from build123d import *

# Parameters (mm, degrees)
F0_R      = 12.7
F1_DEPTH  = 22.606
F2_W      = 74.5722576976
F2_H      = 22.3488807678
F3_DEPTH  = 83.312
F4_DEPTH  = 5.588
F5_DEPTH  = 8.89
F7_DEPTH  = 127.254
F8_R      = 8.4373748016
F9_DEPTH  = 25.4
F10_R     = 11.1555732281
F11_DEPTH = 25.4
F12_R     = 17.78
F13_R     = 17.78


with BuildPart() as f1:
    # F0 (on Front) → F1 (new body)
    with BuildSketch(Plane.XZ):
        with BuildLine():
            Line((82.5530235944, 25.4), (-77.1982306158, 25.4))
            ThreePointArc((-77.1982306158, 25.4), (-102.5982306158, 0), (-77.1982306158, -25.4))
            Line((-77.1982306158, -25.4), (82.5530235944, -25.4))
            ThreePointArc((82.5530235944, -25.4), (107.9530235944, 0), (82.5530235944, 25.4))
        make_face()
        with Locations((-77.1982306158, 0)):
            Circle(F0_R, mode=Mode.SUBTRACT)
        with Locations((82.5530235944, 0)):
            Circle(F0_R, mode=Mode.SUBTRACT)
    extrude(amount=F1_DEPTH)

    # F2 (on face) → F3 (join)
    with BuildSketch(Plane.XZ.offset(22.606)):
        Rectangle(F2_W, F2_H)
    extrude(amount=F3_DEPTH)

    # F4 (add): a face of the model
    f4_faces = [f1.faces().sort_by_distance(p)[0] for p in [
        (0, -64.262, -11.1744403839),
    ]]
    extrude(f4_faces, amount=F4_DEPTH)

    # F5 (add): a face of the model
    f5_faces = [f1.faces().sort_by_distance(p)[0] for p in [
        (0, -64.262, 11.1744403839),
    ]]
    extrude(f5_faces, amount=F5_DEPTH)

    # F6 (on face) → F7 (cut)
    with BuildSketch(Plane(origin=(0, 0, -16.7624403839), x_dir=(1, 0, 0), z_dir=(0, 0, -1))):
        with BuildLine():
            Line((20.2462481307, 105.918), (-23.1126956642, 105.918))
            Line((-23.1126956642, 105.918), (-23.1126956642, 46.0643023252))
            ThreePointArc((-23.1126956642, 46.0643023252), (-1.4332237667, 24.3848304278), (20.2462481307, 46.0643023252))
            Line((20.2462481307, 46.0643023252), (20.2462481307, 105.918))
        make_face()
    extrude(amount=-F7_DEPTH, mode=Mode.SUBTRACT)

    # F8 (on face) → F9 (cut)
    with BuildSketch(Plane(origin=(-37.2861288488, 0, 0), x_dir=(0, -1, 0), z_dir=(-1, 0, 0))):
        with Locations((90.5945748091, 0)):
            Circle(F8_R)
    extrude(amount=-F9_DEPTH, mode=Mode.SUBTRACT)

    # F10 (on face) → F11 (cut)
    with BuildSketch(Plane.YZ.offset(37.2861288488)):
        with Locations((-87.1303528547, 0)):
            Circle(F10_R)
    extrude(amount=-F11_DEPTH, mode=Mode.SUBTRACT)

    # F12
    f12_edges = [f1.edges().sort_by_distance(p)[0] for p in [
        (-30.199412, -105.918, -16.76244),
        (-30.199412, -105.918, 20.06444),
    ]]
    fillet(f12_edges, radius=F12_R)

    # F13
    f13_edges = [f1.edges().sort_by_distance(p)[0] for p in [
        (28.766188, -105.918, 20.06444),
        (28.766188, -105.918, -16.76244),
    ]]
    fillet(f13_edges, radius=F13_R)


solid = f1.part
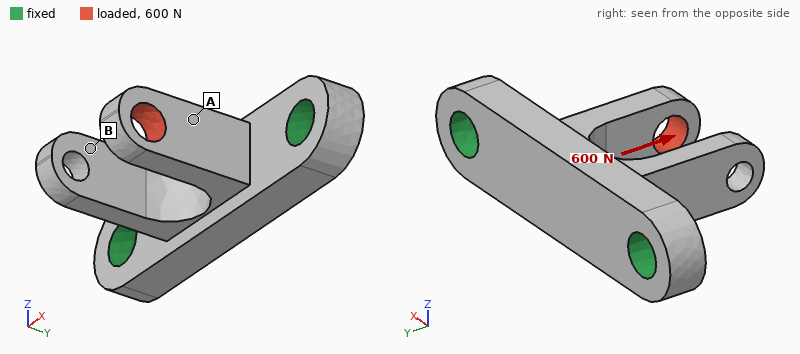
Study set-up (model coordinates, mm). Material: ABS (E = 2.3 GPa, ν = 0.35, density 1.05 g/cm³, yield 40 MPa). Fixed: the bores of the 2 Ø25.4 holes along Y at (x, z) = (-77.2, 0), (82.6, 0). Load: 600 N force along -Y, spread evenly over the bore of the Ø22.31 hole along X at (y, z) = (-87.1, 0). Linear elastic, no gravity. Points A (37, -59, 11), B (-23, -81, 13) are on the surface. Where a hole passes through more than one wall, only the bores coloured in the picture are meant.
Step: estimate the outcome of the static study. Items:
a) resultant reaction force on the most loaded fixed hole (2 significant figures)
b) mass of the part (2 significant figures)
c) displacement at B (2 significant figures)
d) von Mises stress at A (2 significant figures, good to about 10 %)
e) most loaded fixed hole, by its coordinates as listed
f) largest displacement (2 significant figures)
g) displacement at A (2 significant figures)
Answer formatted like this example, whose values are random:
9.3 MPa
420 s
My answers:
450 N
310 g
0.075 mm
0.87 MPa
(82.6, 0)
0.12 mm
0.070 mm
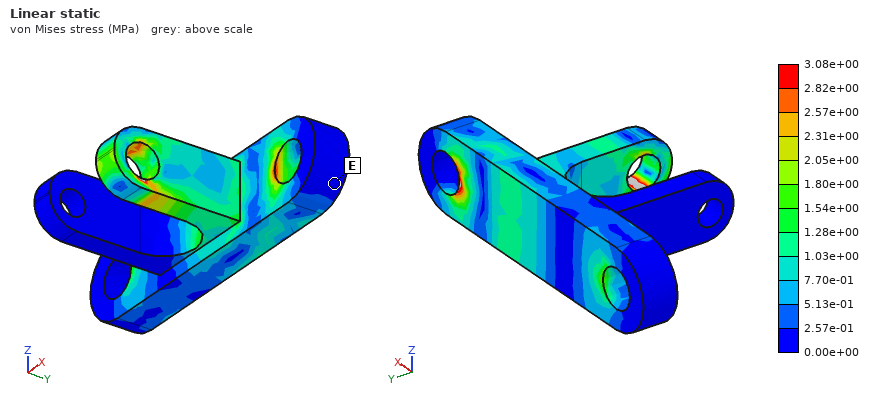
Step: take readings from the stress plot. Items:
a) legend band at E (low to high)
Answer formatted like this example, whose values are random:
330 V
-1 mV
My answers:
0.00e+00 to 2.57e-01 MPa
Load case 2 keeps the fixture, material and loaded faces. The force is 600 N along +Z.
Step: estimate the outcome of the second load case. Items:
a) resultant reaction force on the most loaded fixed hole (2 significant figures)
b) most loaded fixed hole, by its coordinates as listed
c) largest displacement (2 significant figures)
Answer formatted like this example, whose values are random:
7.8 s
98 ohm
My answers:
430 N
(82.6, 0)
1.5 mm
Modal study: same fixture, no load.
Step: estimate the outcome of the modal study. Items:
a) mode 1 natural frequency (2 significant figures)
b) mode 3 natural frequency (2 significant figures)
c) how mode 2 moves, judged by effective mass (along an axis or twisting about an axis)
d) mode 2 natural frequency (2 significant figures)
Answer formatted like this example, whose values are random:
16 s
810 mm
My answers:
650 Hz
780 Hz
along Z
680 Hz
